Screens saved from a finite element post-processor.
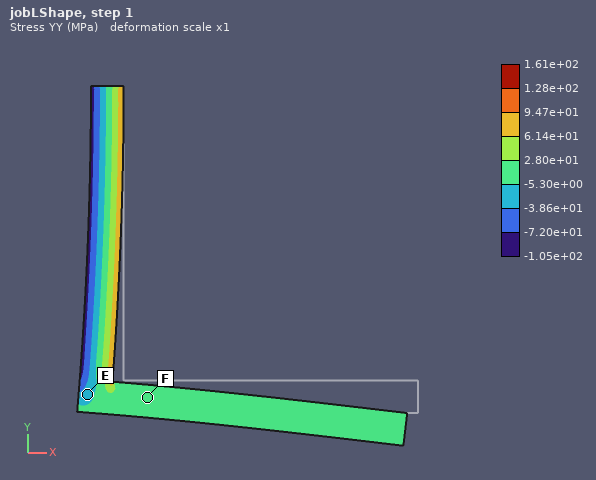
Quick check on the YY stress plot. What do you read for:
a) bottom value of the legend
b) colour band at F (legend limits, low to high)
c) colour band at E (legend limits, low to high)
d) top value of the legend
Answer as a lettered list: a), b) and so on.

a) -1.05e+02 MPa
b) -5.30e+00 to 2.80e+01 MPa
c) -3.86e+01 to -5.30e+00 MPa
d) 1.61e+02 MPa
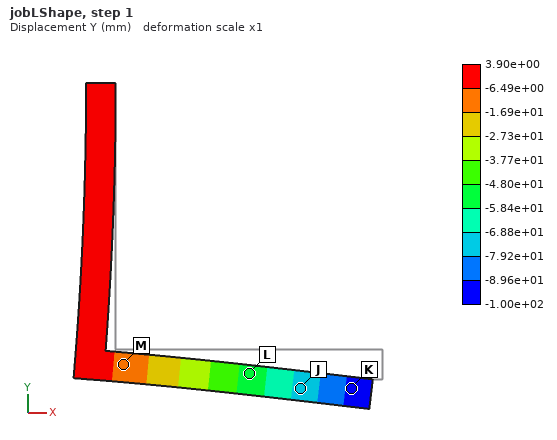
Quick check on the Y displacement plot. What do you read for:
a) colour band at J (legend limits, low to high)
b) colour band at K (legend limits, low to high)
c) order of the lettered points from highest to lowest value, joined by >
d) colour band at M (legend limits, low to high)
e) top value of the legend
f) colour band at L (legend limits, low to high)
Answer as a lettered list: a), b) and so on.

a) -7.92e+01 to -6.88e+01 mm
b) -1.00e+02 to -8.96e+01 mm
c) M > L > J > K
d) -1.69e+01 to -6.49e+00 mm
e) 3.90e+00 mm
f) -5.84e+01 to -4.80e+01 mm
